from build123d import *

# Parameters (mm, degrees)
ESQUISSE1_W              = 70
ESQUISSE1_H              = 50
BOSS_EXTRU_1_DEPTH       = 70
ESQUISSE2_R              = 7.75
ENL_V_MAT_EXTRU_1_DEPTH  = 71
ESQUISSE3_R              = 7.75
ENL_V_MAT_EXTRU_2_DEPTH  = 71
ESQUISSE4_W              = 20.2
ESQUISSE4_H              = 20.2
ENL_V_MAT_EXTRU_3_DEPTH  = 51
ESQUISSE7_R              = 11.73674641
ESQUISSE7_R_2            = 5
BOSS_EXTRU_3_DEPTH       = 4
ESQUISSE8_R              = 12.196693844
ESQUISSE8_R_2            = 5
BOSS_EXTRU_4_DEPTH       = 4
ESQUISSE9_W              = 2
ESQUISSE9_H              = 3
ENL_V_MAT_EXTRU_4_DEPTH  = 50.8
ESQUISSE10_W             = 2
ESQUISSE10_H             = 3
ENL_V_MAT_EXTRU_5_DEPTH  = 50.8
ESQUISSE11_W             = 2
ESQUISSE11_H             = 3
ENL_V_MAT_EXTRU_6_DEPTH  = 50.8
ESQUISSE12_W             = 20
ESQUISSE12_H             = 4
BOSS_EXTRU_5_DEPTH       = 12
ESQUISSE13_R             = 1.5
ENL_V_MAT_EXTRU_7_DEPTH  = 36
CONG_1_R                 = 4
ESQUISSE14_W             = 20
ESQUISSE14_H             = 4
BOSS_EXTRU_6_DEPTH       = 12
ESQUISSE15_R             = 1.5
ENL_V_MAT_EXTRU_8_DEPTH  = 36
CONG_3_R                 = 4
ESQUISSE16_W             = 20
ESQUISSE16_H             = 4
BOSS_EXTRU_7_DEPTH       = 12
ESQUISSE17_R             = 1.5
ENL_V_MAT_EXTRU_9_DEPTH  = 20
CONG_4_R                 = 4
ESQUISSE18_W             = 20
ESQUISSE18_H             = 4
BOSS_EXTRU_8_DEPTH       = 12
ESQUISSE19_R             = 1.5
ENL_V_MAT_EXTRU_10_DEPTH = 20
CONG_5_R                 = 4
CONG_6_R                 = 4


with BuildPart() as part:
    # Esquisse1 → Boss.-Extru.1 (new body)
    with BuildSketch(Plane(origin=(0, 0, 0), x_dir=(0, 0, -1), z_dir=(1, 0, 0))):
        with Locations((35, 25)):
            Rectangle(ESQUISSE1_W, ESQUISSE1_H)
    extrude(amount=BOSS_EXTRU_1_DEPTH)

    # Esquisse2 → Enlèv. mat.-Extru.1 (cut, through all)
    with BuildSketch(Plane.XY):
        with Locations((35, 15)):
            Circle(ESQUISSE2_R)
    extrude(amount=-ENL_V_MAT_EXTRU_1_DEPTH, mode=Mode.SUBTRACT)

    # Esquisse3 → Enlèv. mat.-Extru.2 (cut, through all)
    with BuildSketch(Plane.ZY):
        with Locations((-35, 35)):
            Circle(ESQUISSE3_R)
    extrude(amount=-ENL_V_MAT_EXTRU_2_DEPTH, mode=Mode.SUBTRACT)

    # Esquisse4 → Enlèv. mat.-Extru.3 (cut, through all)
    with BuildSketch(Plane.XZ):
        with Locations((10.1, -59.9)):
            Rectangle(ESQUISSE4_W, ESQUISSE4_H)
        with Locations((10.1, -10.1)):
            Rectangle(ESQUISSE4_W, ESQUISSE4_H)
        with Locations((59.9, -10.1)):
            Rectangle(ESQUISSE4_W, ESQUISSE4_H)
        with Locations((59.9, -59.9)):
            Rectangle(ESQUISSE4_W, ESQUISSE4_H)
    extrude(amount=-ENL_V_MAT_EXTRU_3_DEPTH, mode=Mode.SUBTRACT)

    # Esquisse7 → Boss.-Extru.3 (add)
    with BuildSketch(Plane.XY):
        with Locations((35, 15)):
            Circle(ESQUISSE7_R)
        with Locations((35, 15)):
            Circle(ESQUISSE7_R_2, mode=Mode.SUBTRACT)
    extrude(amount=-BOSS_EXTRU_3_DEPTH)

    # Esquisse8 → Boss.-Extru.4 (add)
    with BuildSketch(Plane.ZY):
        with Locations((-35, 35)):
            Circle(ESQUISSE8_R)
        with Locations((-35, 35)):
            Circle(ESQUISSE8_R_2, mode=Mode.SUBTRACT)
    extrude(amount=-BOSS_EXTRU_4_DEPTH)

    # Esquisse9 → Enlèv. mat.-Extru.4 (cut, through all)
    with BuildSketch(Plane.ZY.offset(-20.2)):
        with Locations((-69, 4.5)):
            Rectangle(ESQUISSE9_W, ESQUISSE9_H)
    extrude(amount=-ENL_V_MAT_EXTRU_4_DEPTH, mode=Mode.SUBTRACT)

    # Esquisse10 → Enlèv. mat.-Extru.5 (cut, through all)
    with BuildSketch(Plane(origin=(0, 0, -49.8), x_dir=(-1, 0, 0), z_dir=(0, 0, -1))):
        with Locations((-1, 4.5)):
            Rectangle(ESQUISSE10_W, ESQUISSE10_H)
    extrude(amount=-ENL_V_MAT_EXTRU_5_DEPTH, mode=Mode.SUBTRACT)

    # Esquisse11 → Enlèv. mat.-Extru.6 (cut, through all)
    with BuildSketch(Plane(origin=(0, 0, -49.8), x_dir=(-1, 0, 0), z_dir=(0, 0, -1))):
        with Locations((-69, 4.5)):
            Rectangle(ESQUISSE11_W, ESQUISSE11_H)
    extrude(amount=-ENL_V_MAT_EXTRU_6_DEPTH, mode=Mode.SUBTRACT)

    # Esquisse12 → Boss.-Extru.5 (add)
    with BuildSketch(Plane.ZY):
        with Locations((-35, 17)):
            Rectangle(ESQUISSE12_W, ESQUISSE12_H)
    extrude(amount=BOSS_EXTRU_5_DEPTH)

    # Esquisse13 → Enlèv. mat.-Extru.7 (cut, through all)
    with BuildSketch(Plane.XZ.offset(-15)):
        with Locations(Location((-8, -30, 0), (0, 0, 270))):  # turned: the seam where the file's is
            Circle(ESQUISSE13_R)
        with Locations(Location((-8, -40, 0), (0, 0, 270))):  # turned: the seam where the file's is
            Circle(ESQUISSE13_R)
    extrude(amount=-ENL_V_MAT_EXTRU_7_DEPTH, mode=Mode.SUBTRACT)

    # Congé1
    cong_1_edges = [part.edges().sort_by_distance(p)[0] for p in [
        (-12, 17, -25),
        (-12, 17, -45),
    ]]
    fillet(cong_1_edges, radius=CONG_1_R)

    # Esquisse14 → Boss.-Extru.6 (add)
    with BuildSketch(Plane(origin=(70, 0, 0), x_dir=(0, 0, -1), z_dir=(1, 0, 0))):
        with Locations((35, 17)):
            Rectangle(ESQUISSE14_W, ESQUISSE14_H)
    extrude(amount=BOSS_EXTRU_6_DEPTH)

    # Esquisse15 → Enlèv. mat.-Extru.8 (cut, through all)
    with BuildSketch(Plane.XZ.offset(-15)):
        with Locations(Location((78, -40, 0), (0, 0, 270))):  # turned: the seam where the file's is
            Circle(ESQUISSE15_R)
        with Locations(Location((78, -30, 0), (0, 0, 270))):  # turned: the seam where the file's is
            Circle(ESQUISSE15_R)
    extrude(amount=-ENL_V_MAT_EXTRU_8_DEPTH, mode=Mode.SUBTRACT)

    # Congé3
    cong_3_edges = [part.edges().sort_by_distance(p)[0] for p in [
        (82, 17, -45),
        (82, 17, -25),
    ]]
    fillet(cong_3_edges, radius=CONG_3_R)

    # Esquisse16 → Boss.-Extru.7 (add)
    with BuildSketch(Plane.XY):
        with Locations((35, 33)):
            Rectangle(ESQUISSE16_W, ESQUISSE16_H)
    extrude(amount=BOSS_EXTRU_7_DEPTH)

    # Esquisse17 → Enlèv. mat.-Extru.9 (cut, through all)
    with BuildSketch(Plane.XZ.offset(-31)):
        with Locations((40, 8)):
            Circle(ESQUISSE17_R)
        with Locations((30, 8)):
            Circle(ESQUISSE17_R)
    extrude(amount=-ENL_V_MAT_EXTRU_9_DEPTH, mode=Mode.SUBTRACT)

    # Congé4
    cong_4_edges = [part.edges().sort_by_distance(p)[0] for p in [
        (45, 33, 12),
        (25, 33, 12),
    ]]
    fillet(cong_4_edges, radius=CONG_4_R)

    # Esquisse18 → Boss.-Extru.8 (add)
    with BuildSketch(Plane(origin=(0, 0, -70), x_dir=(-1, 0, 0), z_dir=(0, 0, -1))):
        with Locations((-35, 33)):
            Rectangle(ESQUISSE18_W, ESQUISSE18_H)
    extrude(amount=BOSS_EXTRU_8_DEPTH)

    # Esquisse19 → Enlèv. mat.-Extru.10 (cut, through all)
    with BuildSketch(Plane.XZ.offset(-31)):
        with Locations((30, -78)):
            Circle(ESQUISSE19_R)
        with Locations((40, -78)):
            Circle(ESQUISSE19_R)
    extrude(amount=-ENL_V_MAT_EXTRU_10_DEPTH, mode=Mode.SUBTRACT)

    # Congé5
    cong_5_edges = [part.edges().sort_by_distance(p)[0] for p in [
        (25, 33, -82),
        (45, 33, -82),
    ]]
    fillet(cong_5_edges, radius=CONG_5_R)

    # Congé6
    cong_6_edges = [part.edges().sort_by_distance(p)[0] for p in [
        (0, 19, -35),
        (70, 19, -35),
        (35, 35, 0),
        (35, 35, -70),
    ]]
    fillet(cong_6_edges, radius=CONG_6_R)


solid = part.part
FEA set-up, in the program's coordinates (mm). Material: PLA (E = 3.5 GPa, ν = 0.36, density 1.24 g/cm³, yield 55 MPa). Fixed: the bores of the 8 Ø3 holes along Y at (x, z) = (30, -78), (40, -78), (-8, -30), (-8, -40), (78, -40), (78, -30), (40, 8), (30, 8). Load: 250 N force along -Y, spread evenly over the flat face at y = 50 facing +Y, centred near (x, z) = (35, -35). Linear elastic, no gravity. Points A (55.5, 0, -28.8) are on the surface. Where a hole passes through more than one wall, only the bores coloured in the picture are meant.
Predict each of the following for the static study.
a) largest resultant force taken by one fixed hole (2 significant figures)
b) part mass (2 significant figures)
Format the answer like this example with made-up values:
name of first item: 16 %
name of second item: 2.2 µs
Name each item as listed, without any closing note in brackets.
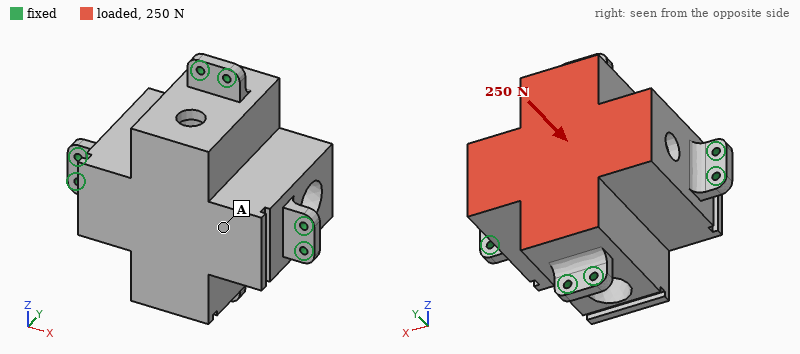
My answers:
largest resultant force taken by one fixed hole: 33 N
part mass: 170 g
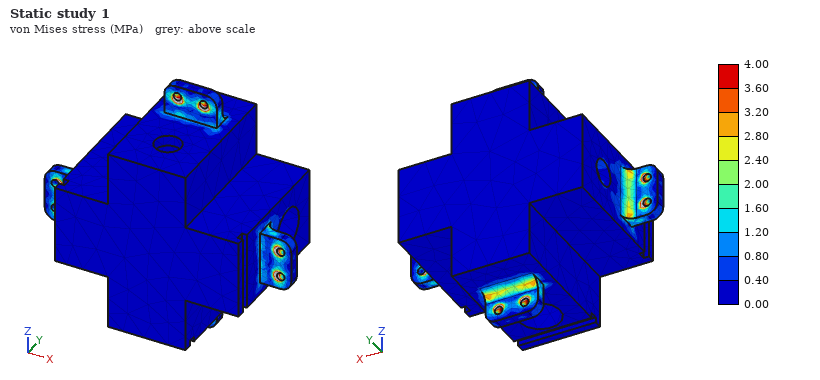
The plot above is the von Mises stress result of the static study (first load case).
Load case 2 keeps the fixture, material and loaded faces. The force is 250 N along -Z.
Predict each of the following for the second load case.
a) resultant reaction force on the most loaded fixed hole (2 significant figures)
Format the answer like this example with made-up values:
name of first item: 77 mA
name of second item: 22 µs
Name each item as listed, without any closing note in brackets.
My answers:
resultant reaction force on the most loaded fixed hole: 66 N
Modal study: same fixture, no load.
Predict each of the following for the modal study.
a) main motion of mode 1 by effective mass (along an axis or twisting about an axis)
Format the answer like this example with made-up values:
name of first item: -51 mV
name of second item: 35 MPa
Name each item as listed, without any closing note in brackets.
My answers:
main motion of mode 1 by effective mass: along Y
